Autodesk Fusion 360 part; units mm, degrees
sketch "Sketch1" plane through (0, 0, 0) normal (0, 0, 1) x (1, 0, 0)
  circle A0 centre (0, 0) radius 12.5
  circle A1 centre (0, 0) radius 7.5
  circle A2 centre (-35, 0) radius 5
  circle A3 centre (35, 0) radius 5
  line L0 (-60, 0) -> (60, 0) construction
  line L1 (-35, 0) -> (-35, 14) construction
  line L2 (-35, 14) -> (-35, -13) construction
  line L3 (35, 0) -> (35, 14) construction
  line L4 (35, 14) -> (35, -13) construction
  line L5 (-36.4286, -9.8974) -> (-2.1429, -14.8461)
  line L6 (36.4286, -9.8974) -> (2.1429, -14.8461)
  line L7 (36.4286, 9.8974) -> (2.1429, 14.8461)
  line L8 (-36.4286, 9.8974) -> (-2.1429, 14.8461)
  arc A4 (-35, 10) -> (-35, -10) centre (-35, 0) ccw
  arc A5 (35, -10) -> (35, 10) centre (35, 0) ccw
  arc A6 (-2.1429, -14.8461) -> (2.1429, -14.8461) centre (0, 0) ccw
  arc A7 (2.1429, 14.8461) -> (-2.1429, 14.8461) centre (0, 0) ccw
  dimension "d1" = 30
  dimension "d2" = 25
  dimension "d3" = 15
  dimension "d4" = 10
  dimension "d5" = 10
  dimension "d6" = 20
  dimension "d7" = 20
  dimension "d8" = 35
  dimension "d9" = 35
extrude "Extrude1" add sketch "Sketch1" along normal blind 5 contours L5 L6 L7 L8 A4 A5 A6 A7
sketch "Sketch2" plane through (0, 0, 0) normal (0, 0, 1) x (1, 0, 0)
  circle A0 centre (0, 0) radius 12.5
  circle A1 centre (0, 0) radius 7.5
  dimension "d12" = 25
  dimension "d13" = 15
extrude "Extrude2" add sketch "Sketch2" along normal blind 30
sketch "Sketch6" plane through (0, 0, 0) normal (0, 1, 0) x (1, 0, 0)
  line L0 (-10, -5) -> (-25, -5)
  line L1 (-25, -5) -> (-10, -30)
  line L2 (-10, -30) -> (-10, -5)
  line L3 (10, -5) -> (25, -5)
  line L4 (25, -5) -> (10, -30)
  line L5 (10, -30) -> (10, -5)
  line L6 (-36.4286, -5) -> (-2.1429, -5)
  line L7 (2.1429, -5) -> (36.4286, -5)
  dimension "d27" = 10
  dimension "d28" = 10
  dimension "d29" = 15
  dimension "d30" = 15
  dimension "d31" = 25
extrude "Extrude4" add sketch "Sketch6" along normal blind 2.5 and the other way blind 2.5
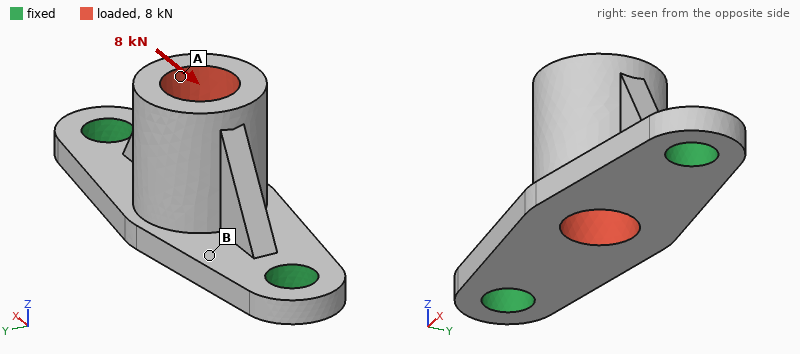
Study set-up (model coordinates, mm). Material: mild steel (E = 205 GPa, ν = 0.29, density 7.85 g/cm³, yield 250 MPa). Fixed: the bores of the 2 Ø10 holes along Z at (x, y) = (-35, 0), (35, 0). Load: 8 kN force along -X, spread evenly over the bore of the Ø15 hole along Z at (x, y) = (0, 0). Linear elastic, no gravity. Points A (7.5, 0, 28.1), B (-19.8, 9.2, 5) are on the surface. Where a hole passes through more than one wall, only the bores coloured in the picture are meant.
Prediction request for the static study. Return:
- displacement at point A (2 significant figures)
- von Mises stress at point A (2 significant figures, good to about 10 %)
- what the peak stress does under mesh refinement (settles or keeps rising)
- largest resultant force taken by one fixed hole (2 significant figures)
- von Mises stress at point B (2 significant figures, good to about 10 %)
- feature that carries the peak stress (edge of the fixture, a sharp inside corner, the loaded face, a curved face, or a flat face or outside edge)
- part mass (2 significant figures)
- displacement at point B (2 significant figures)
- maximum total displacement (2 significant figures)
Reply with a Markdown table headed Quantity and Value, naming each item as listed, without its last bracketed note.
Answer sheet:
| Quantity | Value |
|---|---|
| displacement at point A | 18 µm |
| von Mises stress at point A | 23 MPa |
| what the peak stress does under mesh refinement | keeps rising |
| largest resultant force taken by one fixed hole | 4.4 kN |
| von Mises stress at point B | 50 MPa |
| feature that carries the peak stress | edge of the fixture |
| part mass | 140 g |
| displacement at point B | 5.8 µm |
| maximum total displacement | 19 µm |
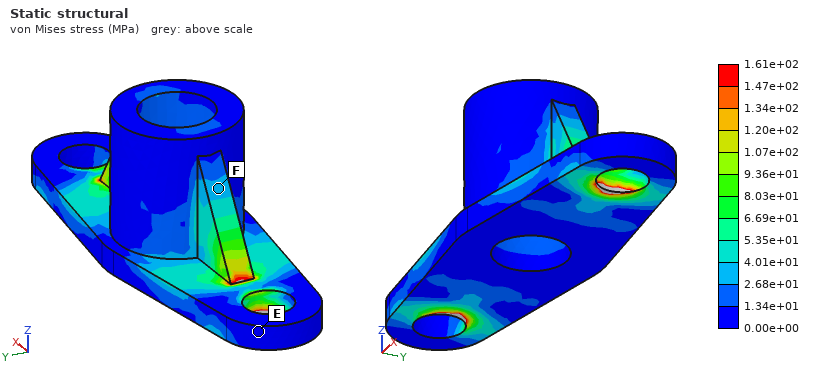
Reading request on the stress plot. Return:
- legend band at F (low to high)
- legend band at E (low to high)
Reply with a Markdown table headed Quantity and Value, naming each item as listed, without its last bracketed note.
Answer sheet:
| Quantity | Value |
|---|---|
| legend band at F | 2.68e+01 to 4.01e+01 MPa |
| legend band at E | 0.00e+00 to 1.34e+01 MPa |
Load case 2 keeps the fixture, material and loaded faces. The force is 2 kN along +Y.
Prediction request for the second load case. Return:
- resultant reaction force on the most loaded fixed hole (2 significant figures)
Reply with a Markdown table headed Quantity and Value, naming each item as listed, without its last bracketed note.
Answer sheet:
| Quantity | Value |
|---|---|
| resultant reaction force on the most loaded fixed hole | 1.0 kN |
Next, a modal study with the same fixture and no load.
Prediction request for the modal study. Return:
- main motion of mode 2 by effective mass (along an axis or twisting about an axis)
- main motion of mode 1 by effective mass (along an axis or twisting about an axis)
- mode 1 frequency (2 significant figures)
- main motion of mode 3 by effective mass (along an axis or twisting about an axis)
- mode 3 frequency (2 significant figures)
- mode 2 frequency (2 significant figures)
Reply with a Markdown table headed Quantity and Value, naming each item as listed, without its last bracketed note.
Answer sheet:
| Quantity | Value |
|---|---|
| main motion of mode 2 by effective mass | along Z |
| main motion of mode 1 by effective mass | along Y |
| mode 1 frequency | 3200 Hz |
| main motion of mode 3 by effective mass | along X |
| mode 3 frequency | 12 kHz |
| mode 2 frequency | 7300 Hz |
